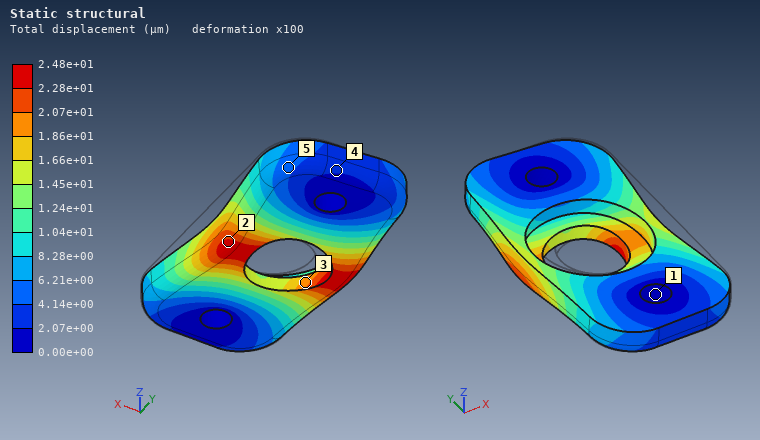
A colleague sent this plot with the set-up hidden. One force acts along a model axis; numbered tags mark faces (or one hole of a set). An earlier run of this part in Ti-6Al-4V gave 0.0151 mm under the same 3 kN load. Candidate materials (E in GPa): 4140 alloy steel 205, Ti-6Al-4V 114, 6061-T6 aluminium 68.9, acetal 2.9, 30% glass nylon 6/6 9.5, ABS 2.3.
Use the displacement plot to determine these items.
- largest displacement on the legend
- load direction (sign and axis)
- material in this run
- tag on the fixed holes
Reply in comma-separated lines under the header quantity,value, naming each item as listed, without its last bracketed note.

quantity,value
largest displacement on the legend,2.48e+01 µm
load direction,-X
material in this run,6061-T6 aluminium
tag on the fixed holes,1
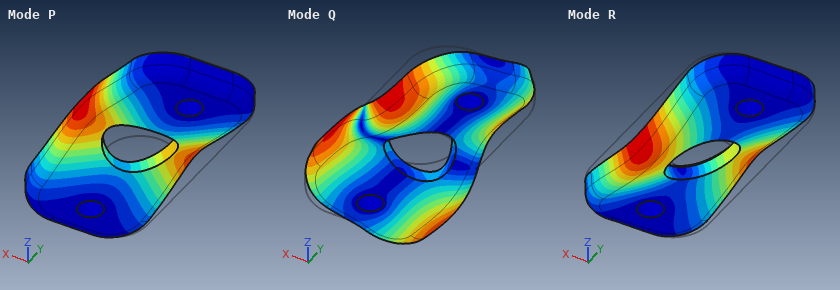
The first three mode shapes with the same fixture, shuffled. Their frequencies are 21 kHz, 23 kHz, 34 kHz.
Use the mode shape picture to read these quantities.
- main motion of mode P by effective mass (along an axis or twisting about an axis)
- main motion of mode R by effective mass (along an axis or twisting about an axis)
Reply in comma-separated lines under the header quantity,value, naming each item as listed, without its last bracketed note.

quantity,value
main motion of mode P by effective mass,along Z
main motion of mode R by effective mass,twisting about Y
